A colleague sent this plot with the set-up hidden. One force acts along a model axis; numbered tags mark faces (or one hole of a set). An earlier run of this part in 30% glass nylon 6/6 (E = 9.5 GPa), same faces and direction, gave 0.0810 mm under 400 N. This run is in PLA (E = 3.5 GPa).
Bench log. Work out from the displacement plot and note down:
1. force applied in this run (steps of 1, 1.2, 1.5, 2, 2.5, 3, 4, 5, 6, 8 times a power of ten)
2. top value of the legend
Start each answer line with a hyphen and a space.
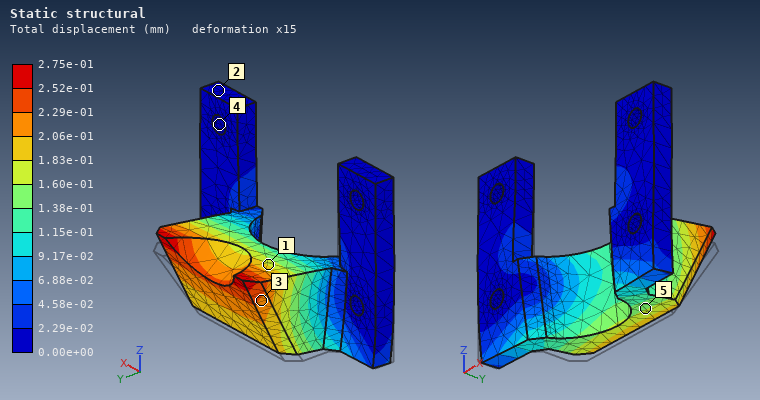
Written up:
- 500 N
- 2.75e-01 mm
